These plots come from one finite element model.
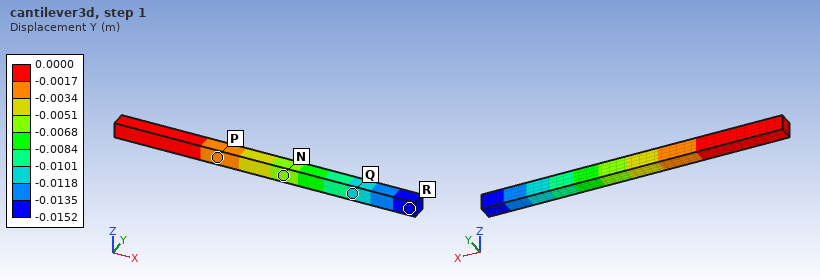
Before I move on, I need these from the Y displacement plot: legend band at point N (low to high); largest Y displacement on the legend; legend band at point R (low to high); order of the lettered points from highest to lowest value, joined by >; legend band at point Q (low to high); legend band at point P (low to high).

-0.0068 to -0.0051 m
0.0000 m
-0.0152 to -0.0135 m
P > N > Q > R
-0.0118 to -0.0101 m
-0.0034 to -0.0017 m
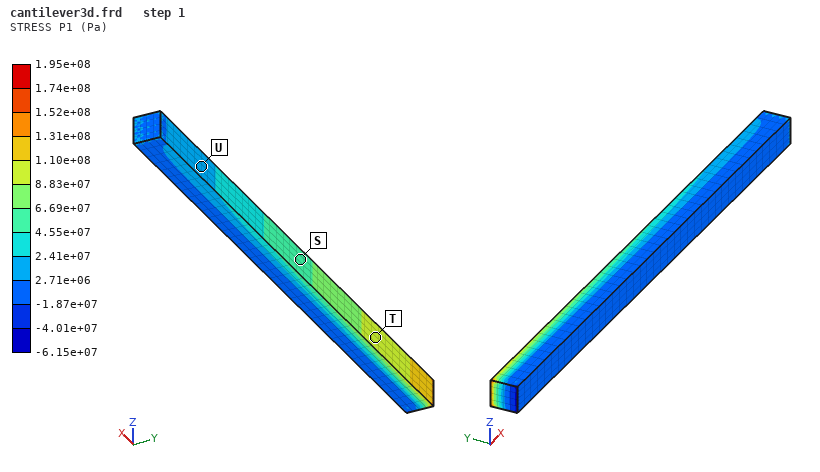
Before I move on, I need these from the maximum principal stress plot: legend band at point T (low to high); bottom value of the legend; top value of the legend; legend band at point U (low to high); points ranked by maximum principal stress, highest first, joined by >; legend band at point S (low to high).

8.83e+07 to 1.10e+08 Pa
-6.15e+07 Pa
1.95e+08 Pa
2.71e+06 to 2.41e+07 Pa
T > S > U
4.55e+07 to 6.69e+07 Pa
